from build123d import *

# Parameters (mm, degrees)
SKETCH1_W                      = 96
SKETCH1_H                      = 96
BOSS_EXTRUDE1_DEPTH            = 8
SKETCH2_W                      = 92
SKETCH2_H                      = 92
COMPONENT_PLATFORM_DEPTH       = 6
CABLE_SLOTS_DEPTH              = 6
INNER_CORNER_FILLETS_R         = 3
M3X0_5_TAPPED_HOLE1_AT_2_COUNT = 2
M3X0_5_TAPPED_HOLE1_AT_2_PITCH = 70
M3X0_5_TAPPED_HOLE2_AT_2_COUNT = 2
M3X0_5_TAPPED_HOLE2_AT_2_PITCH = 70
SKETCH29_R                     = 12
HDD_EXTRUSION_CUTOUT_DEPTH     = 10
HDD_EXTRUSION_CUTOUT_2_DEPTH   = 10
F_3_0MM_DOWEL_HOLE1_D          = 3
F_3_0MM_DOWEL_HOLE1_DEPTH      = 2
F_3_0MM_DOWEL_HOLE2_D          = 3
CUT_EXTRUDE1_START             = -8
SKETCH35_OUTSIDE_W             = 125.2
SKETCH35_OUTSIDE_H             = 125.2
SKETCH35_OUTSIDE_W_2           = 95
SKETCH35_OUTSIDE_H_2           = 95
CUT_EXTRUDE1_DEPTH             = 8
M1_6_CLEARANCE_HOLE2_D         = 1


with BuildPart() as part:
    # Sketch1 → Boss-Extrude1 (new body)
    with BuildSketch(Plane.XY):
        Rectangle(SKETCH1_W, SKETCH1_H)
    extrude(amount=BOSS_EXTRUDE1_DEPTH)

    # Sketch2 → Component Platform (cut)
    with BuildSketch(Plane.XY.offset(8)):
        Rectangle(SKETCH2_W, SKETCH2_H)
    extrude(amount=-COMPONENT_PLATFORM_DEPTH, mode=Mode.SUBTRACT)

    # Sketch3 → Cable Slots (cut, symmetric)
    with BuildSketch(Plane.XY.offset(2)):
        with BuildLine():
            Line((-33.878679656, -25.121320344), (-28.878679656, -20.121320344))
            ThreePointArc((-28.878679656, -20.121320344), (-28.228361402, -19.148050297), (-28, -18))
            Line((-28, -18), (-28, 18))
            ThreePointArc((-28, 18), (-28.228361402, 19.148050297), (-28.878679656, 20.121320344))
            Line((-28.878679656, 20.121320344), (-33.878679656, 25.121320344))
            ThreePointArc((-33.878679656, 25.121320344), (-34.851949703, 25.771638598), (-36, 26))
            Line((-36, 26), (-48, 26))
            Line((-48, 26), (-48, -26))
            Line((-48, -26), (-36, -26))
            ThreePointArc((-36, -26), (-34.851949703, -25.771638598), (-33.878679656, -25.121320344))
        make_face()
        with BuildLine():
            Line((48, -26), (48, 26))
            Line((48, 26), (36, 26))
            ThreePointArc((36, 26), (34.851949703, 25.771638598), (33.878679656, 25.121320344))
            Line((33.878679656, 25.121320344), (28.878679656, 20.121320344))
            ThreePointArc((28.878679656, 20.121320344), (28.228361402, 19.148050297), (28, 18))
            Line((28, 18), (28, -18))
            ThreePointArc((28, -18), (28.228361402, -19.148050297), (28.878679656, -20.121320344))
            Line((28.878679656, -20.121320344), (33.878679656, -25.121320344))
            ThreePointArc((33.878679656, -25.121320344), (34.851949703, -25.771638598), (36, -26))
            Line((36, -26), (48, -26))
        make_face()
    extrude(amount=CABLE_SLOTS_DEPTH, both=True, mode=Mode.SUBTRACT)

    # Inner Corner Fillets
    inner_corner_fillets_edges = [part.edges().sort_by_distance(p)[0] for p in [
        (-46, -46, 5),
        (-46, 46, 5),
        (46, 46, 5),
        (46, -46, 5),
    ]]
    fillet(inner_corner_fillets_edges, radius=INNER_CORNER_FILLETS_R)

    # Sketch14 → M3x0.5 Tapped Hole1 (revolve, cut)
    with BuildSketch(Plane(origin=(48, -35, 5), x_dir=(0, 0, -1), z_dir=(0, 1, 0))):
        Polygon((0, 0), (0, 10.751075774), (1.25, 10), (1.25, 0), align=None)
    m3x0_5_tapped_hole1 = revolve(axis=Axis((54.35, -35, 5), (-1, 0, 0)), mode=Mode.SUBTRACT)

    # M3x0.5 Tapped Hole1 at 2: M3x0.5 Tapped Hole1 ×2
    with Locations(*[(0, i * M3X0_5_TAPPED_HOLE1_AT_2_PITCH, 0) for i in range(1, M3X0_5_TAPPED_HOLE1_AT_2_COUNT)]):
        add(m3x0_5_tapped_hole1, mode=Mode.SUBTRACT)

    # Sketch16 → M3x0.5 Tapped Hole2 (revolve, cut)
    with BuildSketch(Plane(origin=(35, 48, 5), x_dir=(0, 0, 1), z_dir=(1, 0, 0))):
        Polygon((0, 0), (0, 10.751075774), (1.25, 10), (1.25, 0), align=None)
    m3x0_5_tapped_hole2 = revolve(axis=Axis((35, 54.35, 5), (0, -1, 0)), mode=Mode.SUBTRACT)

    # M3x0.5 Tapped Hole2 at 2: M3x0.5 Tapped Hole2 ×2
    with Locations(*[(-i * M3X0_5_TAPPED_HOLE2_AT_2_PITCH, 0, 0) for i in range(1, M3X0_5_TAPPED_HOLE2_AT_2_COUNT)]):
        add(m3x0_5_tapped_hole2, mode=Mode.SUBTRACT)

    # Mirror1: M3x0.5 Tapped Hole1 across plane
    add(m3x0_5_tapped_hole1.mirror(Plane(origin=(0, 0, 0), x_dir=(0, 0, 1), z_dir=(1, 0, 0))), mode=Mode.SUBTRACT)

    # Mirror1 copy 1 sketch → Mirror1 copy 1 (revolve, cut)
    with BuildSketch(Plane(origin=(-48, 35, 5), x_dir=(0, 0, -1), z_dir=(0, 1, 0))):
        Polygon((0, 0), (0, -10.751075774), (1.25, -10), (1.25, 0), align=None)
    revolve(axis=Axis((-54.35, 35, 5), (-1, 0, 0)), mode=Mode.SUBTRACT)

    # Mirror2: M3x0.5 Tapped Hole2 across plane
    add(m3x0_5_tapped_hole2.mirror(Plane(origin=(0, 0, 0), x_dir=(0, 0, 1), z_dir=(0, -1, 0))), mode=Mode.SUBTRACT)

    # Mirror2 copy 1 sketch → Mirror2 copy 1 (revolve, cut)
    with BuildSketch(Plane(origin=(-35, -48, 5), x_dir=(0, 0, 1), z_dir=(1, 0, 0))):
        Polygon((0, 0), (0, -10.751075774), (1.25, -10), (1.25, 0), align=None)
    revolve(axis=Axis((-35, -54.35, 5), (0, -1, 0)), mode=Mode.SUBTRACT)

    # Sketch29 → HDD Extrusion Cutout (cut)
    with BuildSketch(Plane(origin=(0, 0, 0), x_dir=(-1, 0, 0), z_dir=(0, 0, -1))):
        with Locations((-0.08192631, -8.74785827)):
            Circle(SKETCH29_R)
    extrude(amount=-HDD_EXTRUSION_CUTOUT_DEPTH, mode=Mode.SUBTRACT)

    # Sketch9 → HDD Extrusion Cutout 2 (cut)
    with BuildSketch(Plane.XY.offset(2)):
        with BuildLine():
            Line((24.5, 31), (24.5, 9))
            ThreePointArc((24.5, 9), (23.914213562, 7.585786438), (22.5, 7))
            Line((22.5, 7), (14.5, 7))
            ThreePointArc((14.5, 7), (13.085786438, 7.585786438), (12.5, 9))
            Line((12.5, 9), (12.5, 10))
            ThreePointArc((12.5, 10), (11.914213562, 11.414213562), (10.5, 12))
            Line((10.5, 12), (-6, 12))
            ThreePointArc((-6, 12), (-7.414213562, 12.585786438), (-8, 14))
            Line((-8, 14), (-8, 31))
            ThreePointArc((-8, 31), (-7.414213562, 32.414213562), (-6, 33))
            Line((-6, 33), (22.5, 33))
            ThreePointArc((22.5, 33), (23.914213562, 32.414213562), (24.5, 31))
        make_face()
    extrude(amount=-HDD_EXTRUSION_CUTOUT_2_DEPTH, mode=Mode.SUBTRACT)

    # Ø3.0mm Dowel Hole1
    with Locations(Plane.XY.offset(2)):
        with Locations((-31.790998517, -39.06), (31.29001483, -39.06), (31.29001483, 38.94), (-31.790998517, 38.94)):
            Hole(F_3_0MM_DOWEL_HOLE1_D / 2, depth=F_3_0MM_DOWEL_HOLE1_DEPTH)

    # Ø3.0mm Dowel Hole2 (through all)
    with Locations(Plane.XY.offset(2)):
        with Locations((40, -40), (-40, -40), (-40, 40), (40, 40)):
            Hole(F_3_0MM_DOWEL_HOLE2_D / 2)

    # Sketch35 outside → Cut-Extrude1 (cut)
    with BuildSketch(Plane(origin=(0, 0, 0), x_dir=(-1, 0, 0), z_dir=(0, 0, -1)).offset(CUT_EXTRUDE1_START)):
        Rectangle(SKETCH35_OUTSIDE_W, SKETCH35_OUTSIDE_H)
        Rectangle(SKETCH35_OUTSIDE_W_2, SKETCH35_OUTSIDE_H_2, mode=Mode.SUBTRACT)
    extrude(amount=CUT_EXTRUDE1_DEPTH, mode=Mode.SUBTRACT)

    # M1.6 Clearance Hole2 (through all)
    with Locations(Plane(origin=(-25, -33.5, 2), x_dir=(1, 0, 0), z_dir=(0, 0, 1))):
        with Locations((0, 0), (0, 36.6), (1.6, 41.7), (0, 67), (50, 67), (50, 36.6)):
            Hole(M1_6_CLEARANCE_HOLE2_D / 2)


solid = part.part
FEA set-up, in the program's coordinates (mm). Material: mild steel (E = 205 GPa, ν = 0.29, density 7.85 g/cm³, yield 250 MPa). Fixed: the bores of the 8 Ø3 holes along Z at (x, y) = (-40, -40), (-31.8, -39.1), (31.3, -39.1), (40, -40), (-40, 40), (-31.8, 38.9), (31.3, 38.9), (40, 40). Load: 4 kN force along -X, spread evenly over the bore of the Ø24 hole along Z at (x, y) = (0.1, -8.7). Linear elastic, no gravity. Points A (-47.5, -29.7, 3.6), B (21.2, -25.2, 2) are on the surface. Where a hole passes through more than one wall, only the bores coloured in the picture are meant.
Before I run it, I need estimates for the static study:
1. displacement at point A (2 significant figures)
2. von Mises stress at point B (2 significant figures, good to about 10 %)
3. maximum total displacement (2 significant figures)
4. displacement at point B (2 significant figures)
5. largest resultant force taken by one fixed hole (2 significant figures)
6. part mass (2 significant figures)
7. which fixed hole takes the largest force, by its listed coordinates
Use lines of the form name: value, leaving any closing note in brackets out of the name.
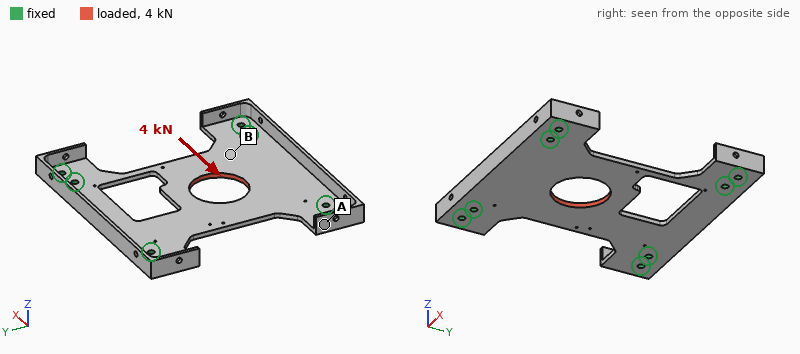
displacement at point A: 3.0 µm
von Mises stress at point B: 27 MPa
maximum total displacement: 20 µm
displacement at point B: 4.8 µm
largest resultant force taken by one fixed hole: 1.3 kN
part mass: 110 g
which fixed hole takes the largest force, by its listed coordinates: (-31.8, -39.1)
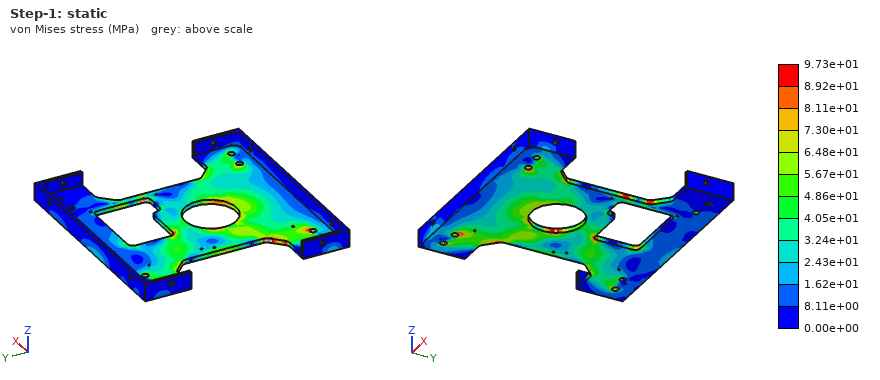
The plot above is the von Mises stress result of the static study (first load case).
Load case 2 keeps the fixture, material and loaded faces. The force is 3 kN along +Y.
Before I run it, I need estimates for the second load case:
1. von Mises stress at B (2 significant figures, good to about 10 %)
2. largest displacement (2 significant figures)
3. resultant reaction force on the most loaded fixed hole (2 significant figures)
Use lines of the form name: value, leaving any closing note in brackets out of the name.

von Mises stress at B: 26 MPa
largest displacement: 11 µm
resultant reaction force on the most loaded fixed hole: 1.1 kN
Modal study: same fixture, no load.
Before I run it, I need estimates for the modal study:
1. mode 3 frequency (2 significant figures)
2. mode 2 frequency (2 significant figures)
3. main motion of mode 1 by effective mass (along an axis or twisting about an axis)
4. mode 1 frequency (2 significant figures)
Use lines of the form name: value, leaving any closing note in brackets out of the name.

mode 3 frequency: 3300 Hz
mode 2 frequency: 2400 Hz
main motion of mode 1 by effective mass: along Z
mode 1 frequency: 1400 Hz
